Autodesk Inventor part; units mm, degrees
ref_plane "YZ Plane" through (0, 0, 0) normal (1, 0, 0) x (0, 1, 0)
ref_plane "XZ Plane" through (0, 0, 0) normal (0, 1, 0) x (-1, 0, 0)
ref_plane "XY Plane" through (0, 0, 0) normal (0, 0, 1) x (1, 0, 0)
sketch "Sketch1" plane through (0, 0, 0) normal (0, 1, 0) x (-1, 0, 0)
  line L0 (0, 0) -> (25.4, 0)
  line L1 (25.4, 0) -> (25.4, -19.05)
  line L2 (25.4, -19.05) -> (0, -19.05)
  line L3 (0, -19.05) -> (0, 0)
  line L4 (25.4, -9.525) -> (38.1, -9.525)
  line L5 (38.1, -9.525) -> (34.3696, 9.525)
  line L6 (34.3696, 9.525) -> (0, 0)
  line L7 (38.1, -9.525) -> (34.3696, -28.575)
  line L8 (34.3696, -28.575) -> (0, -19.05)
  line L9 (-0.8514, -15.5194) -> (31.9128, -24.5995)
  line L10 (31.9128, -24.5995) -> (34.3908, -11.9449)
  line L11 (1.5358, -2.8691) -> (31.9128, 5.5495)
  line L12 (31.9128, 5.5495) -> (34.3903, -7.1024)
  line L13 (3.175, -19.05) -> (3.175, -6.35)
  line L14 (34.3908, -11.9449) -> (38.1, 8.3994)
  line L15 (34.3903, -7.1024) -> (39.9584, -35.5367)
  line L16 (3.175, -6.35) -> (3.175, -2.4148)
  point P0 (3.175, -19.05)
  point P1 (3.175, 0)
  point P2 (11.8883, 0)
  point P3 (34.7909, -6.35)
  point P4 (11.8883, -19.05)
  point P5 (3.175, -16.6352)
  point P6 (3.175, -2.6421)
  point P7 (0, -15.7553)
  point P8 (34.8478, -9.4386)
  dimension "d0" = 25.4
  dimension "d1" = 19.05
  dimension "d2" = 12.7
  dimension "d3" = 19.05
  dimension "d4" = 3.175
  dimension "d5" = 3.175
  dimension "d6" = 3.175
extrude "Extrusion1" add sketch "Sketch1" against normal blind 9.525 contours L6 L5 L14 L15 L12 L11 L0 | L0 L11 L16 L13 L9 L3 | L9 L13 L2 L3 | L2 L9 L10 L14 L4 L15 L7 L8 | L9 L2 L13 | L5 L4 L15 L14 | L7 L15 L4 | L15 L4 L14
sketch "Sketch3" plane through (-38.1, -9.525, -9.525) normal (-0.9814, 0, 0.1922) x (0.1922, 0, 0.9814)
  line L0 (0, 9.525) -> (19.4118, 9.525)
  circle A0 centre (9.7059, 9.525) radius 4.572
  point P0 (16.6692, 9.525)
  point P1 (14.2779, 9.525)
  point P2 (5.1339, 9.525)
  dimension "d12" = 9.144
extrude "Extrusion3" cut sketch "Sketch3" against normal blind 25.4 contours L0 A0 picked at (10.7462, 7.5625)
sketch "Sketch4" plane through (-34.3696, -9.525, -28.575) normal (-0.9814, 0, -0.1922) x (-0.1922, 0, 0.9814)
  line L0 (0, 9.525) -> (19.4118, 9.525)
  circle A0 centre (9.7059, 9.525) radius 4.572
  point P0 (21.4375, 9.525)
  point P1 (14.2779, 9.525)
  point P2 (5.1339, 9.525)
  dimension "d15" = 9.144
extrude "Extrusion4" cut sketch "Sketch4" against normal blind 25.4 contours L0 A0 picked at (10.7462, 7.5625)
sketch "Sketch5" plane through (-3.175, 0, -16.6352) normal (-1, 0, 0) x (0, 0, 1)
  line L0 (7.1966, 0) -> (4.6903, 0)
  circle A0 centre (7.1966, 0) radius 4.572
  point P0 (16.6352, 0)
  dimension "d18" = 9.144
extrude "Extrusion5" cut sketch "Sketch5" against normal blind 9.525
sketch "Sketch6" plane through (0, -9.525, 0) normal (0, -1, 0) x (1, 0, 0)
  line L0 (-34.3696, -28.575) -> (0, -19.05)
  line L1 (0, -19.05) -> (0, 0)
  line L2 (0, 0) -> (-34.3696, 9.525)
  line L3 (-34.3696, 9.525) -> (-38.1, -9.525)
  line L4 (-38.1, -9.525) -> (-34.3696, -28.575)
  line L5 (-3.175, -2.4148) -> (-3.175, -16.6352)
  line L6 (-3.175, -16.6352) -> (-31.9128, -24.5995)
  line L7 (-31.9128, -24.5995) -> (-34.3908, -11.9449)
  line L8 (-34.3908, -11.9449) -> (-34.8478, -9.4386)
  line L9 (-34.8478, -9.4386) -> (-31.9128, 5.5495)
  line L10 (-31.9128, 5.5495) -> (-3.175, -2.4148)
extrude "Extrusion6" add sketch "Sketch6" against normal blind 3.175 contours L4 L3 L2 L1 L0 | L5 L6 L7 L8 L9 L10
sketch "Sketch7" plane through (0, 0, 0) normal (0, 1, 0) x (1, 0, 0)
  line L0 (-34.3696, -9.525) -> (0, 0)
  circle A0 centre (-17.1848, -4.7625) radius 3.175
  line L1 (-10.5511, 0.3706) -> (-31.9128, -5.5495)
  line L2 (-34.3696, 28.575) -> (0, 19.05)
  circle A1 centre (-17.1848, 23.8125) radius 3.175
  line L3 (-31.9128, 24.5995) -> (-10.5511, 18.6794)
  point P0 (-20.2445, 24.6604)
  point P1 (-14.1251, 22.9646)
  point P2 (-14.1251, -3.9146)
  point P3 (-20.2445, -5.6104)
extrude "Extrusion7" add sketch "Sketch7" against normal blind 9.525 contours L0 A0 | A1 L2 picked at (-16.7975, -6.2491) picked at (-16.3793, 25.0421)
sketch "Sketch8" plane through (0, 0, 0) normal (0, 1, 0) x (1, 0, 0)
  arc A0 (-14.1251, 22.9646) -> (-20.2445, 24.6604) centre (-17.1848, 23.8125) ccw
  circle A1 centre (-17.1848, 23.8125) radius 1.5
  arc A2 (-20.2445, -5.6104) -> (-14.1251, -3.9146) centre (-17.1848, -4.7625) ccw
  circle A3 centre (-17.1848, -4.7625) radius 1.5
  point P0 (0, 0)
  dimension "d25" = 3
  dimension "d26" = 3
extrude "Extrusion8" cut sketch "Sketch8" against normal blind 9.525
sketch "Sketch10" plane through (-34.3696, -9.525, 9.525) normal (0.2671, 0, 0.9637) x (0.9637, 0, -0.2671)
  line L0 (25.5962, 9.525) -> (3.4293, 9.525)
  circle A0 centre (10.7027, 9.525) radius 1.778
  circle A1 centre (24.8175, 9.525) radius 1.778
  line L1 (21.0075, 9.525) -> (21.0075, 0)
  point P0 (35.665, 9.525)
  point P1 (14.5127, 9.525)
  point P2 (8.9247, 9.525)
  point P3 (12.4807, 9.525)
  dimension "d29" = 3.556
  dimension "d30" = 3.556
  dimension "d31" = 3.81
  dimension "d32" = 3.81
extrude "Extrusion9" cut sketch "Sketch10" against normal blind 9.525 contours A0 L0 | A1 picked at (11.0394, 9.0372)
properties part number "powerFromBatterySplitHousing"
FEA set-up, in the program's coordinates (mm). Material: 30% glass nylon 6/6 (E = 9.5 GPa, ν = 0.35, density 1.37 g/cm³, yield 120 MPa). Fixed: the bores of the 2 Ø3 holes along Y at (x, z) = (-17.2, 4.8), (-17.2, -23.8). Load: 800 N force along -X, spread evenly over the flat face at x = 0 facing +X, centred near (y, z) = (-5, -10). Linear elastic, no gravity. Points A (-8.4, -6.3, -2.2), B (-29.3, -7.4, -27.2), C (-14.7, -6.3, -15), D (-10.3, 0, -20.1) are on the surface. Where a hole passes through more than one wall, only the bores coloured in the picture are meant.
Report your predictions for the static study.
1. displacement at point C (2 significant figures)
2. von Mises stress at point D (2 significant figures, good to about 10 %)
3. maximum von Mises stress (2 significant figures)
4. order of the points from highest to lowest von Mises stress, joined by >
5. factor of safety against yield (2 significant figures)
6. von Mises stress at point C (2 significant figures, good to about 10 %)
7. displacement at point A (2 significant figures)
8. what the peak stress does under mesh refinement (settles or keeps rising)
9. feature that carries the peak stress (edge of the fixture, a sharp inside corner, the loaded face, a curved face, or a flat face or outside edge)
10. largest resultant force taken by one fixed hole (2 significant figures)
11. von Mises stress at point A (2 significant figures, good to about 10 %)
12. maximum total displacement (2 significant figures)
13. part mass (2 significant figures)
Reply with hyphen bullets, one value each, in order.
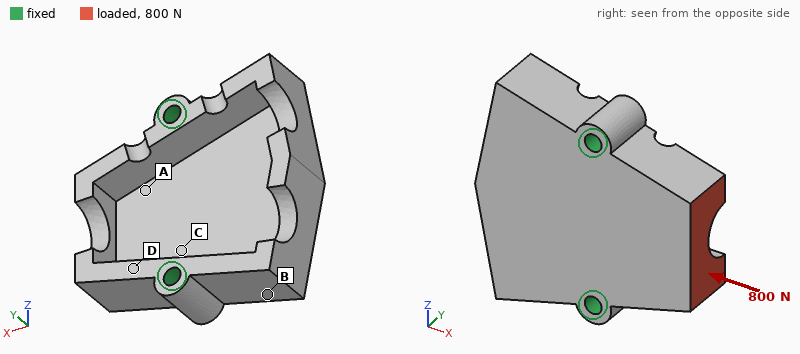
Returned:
- 8.7 µm
- 13 MPa
- 38 MPa
- D > A > C > B
- 3.1
- 4.8 MPa
- 11 µm
- settles
- a curved face
- 420 N
- 8.9 MPa
- 52 µm
- 7.6 g
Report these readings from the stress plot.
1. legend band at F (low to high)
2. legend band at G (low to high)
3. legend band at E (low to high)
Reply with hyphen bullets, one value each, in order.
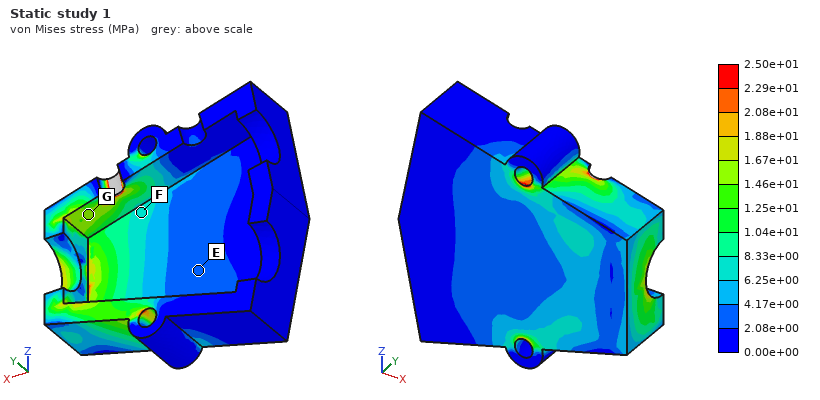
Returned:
- 6.25e+00 to 8.33e+00 MPa
- 1.46e+01 to 1.67e+01 MPa
- 2.08e+00 to 4.17e+00 MPa
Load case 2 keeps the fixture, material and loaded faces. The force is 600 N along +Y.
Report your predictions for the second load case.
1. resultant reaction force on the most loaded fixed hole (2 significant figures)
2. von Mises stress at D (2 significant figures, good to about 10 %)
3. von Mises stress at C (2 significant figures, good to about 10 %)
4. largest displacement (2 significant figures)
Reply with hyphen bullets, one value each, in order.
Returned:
- 340 N
- 58 MPa
- 12 MPa
- 0.31 mm
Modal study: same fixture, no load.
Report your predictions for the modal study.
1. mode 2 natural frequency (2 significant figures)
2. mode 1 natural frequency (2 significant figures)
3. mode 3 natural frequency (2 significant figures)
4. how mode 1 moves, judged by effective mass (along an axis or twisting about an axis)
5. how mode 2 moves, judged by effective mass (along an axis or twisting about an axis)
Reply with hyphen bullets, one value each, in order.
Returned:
- 7800 Hz
- 4800 Hz
- 8500 Hz
- along Y
- along Y
